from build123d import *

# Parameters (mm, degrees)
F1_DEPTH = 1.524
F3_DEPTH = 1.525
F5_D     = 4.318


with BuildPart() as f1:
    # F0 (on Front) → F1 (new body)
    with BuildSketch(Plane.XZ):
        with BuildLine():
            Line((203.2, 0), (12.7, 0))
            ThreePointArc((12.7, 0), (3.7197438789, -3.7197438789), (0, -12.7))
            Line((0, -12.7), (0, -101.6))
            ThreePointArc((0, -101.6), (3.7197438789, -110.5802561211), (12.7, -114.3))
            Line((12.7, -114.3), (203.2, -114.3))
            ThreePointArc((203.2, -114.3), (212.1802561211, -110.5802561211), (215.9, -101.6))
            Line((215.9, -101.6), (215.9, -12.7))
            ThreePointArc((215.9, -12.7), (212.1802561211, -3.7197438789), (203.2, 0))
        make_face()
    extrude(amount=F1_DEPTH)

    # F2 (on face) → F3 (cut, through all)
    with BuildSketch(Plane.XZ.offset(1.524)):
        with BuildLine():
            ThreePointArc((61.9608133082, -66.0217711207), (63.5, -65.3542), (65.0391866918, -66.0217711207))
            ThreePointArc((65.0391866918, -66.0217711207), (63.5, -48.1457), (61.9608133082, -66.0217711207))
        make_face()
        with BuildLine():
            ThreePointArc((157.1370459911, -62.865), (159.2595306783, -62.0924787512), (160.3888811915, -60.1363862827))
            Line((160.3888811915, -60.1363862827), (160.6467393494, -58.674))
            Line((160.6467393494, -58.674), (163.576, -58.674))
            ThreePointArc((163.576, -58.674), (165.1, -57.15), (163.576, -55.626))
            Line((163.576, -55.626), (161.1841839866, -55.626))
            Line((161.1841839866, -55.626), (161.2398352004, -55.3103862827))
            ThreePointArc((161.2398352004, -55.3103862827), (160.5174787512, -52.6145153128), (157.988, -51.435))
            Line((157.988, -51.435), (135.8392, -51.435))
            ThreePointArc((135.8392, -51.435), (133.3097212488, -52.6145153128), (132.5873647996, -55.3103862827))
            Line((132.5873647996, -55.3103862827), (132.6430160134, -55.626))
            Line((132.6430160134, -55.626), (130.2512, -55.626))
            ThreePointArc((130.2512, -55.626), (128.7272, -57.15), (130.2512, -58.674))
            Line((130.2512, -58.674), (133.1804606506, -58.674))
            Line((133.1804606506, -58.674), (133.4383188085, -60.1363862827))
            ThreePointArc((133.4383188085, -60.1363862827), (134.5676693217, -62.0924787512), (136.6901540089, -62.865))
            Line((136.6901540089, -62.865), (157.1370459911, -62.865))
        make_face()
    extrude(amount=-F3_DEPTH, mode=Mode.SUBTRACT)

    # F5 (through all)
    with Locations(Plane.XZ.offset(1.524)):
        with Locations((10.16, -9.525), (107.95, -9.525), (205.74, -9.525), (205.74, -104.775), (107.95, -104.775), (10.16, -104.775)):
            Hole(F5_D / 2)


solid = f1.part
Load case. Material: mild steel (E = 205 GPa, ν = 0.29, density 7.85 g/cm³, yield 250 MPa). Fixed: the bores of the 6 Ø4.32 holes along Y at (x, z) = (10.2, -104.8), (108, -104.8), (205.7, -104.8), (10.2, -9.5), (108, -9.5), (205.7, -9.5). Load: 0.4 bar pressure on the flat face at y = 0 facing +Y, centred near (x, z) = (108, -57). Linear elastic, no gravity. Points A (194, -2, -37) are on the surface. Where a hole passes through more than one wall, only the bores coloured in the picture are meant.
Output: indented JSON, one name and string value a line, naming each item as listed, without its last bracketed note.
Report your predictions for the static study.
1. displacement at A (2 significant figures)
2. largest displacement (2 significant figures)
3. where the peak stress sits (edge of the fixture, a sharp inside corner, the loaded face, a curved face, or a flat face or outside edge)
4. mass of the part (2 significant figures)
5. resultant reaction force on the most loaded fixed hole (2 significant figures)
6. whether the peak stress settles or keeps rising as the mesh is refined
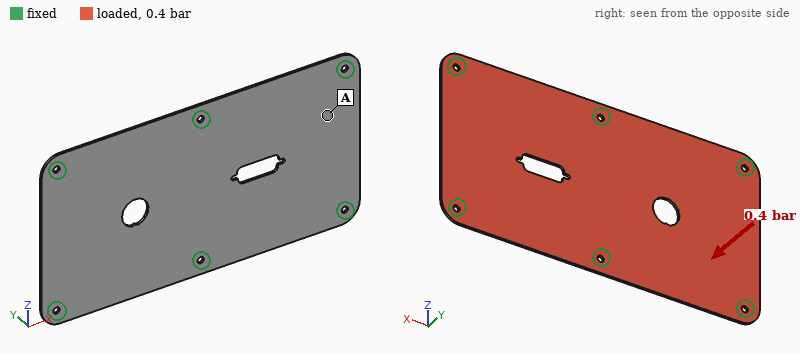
{
  "displacement at A": "0.20 mm",
  "largest displacement": "0.41 mm",
  "where the peak stress sits": "edge of the fixture",
  "mass of the part": "290 g",
  "resultant reaction force on the most loaded fixed hole": "230 N",
  "whether the peak stress settles or keeps rising as the mesh is refined": "keeps rising"
}
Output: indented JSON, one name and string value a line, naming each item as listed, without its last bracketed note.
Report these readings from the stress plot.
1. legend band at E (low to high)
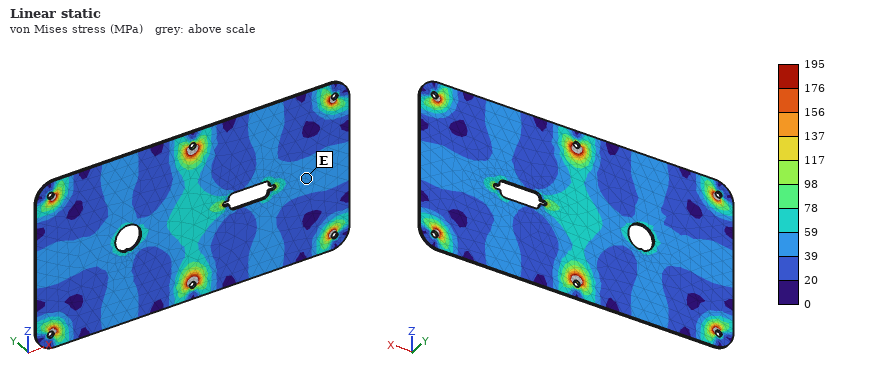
{
  "legend band at E": "39 to 59 MPa"
}
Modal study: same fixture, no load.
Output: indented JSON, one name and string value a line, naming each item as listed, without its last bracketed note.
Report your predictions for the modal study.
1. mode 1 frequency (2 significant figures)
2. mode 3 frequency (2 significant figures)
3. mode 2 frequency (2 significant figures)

{
  "mode 1 frequency": "570 Hz",
  "mode 3 frequency": "930 Hz",
  "mode 2 frequency": "580 Hz"
}
